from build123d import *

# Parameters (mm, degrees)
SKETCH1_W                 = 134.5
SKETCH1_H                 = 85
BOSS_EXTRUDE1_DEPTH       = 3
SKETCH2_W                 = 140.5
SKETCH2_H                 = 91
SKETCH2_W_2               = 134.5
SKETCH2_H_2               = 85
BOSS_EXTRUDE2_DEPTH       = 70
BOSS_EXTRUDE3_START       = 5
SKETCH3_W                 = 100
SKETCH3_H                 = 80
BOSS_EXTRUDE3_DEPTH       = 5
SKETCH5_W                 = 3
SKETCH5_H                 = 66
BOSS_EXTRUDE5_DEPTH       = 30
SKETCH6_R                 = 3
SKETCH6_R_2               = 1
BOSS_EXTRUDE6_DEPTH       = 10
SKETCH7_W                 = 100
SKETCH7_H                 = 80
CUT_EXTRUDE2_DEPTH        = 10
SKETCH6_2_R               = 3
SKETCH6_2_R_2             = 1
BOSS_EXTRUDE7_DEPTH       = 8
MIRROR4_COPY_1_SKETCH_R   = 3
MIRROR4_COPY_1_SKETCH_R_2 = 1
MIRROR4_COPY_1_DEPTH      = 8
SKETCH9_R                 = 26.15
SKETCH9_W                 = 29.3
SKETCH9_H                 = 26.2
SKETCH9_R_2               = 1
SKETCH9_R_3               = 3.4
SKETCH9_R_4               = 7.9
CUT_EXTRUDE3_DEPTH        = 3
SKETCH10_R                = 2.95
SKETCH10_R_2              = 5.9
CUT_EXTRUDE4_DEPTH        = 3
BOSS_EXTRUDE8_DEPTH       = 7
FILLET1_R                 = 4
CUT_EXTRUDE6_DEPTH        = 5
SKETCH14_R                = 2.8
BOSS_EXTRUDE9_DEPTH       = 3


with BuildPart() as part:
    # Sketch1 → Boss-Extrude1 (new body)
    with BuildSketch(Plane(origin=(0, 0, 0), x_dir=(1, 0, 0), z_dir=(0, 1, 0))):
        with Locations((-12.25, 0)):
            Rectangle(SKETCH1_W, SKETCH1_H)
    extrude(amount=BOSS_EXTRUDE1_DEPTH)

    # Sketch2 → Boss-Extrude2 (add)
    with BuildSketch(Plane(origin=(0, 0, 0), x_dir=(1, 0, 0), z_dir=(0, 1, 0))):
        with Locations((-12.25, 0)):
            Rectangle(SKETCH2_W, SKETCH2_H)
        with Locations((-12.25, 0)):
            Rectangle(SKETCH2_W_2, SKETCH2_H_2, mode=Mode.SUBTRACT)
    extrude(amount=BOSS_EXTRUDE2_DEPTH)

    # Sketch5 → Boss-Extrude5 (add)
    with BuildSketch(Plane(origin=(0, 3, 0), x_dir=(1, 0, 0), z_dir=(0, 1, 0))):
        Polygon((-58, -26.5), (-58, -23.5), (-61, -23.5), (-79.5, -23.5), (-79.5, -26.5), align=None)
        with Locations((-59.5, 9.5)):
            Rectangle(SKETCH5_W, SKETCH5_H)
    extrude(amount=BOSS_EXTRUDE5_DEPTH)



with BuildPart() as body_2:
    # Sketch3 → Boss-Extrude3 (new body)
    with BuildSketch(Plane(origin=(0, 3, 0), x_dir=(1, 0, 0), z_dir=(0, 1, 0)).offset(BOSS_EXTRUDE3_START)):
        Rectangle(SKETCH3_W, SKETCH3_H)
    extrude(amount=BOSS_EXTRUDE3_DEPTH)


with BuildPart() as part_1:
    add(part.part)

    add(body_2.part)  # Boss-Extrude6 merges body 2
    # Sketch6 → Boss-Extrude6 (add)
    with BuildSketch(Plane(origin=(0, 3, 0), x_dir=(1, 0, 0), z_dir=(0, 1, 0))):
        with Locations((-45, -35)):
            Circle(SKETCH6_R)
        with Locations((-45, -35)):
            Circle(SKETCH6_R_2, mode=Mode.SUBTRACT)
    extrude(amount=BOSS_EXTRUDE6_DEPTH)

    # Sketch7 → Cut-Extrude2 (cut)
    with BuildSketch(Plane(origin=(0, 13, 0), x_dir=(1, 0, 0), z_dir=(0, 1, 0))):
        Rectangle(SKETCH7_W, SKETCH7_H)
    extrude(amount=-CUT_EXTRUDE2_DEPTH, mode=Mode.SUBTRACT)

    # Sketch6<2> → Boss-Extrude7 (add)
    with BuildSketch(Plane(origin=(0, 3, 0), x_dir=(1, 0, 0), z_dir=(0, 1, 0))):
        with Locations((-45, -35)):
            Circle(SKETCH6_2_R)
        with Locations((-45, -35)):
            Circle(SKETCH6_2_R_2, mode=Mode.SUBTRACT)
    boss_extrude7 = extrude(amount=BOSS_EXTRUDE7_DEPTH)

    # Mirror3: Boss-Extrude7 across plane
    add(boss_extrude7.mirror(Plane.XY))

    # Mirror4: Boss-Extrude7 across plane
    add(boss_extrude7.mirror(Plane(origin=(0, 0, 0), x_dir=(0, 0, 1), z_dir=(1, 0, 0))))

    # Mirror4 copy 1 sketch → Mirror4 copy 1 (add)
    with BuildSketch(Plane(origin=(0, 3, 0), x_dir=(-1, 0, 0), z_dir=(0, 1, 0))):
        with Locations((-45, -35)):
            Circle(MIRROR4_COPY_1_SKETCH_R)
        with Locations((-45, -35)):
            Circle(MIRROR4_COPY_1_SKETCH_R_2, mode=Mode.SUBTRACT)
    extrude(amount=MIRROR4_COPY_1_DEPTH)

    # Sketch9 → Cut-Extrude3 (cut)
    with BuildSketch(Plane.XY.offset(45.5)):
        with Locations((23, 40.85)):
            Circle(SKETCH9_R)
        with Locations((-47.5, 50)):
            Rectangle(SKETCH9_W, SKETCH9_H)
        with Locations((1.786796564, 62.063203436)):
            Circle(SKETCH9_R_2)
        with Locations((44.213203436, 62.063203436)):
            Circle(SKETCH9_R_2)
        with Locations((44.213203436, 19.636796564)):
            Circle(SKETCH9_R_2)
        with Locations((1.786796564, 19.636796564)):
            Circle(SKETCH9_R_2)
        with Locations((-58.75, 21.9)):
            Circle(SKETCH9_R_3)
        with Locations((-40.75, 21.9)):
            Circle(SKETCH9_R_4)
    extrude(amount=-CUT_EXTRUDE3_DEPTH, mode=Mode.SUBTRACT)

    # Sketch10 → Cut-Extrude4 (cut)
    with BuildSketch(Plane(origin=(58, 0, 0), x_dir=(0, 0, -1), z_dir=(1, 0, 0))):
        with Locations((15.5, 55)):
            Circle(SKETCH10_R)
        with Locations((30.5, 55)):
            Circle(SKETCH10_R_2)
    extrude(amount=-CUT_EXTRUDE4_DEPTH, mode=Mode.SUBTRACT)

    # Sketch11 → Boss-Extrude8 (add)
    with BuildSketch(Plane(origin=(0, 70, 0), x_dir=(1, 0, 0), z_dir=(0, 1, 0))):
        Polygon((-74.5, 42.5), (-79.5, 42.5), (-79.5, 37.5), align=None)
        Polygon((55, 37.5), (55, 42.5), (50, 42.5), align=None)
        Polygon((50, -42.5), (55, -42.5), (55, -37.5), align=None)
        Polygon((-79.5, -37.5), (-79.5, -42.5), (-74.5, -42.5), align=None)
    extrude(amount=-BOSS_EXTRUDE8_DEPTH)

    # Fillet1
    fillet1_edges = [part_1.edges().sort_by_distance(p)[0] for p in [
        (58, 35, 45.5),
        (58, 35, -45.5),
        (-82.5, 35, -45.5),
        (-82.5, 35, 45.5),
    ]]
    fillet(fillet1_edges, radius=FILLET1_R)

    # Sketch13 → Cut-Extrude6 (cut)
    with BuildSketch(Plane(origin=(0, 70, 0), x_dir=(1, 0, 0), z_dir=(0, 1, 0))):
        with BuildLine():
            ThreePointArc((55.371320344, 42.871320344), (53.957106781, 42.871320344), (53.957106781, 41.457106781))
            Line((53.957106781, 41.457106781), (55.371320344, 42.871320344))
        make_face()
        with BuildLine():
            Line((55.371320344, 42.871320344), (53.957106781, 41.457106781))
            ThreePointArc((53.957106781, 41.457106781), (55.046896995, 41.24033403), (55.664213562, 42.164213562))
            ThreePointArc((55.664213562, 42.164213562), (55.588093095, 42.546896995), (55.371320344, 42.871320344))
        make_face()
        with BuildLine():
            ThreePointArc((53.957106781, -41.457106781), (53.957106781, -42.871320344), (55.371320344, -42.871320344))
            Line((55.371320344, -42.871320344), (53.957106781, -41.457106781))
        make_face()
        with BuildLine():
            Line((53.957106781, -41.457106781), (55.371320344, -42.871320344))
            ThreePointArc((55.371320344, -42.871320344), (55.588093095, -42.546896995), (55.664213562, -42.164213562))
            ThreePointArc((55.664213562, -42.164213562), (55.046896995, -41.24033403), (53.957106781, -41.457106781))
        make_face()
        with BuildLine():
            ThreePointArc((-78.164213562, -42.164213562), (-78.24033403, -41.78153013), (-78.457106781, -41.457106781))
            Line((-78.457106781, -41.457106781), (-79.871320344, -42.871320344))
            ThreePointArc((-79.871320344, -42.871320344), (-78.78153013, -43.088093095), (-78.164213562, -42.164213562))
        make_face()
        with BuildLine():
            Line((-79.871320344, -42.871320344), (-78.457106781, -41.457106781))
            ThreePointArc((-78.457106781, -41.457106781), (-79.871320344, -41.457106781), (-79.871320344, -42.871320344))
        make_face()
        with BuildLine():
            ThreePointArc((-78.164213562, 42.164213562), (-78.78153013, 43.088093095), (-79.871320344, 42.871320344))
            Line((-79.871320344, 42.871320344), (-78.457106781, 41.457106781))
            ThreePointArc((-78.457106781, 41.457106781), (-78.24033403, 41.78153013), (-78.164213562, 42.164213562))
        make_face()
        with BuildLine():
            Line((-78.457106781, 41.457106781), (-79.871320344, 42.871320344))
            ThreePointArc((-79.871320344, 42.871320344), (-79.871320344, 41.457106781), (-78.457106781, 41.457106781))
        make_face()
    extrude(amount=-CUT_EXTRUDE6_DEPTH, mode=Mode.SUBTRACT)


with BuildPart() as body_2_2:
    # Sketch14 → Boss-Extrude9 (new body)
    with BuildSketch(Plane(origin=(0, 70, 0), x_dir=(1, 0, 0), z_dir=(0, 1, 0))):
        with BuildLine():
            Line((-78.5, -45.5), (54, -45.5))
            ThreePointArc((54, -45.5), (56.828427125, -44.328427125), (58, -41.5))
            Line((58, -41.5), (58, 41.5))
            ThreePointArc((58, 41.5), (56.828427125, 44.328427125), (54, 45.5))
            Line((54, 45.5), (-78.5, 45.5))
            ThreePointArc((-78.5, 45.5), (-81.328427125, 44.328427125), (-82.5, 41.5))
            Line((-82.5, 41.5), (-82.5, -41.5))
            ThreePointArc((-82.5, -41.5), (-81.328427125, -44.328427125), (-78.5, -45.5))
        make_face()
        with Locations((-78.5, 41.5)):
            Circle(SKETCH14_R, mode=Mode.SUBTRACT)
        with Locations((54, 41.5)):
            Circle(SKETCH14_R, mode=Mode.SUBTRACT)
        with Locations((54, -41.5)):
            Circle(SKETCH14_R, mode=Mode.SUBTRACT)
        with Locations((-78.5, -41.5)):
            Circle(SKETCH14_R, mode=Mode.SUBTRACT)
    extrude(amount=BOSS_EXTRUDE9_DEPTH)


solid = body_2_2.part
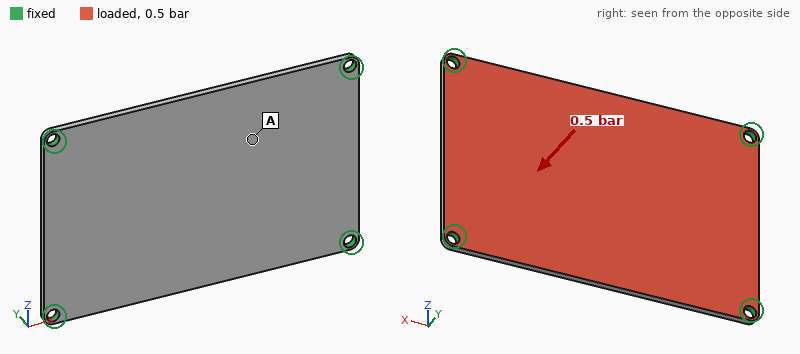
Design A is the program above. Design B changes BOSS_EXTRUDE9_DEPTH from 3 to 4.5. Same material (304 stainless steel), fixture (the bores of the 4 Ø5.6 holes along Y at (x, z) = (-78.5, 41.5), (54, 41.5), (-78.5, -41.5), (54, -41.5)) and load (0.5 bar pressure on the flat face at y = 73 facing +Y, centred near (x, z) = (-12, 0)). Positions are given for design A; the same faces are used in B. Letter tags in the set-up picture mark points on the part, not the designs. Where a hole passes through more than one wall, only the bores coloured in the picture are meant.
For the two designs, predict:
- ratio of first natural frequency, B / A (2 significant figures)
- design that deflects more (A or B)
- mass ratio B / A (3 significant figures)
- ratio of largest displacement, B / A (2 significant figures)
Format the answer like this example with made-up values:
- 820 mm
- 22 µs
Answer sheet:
- 1.5
- A
- 1.50
- 0.31
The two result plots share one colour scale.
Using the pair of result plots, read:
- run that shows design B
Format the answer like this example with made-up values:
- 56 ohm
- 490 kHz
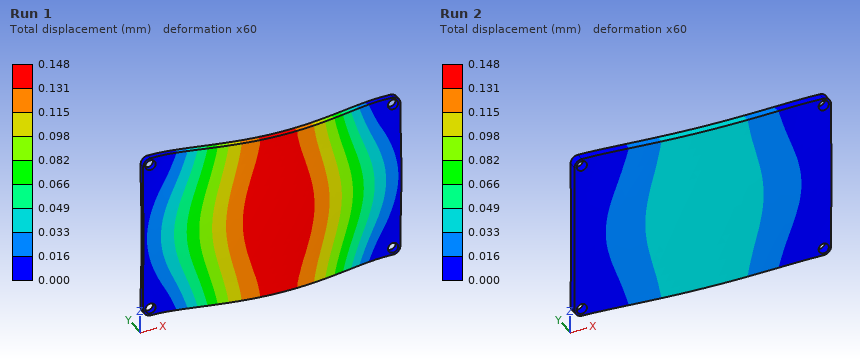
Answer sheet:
- Run 2
